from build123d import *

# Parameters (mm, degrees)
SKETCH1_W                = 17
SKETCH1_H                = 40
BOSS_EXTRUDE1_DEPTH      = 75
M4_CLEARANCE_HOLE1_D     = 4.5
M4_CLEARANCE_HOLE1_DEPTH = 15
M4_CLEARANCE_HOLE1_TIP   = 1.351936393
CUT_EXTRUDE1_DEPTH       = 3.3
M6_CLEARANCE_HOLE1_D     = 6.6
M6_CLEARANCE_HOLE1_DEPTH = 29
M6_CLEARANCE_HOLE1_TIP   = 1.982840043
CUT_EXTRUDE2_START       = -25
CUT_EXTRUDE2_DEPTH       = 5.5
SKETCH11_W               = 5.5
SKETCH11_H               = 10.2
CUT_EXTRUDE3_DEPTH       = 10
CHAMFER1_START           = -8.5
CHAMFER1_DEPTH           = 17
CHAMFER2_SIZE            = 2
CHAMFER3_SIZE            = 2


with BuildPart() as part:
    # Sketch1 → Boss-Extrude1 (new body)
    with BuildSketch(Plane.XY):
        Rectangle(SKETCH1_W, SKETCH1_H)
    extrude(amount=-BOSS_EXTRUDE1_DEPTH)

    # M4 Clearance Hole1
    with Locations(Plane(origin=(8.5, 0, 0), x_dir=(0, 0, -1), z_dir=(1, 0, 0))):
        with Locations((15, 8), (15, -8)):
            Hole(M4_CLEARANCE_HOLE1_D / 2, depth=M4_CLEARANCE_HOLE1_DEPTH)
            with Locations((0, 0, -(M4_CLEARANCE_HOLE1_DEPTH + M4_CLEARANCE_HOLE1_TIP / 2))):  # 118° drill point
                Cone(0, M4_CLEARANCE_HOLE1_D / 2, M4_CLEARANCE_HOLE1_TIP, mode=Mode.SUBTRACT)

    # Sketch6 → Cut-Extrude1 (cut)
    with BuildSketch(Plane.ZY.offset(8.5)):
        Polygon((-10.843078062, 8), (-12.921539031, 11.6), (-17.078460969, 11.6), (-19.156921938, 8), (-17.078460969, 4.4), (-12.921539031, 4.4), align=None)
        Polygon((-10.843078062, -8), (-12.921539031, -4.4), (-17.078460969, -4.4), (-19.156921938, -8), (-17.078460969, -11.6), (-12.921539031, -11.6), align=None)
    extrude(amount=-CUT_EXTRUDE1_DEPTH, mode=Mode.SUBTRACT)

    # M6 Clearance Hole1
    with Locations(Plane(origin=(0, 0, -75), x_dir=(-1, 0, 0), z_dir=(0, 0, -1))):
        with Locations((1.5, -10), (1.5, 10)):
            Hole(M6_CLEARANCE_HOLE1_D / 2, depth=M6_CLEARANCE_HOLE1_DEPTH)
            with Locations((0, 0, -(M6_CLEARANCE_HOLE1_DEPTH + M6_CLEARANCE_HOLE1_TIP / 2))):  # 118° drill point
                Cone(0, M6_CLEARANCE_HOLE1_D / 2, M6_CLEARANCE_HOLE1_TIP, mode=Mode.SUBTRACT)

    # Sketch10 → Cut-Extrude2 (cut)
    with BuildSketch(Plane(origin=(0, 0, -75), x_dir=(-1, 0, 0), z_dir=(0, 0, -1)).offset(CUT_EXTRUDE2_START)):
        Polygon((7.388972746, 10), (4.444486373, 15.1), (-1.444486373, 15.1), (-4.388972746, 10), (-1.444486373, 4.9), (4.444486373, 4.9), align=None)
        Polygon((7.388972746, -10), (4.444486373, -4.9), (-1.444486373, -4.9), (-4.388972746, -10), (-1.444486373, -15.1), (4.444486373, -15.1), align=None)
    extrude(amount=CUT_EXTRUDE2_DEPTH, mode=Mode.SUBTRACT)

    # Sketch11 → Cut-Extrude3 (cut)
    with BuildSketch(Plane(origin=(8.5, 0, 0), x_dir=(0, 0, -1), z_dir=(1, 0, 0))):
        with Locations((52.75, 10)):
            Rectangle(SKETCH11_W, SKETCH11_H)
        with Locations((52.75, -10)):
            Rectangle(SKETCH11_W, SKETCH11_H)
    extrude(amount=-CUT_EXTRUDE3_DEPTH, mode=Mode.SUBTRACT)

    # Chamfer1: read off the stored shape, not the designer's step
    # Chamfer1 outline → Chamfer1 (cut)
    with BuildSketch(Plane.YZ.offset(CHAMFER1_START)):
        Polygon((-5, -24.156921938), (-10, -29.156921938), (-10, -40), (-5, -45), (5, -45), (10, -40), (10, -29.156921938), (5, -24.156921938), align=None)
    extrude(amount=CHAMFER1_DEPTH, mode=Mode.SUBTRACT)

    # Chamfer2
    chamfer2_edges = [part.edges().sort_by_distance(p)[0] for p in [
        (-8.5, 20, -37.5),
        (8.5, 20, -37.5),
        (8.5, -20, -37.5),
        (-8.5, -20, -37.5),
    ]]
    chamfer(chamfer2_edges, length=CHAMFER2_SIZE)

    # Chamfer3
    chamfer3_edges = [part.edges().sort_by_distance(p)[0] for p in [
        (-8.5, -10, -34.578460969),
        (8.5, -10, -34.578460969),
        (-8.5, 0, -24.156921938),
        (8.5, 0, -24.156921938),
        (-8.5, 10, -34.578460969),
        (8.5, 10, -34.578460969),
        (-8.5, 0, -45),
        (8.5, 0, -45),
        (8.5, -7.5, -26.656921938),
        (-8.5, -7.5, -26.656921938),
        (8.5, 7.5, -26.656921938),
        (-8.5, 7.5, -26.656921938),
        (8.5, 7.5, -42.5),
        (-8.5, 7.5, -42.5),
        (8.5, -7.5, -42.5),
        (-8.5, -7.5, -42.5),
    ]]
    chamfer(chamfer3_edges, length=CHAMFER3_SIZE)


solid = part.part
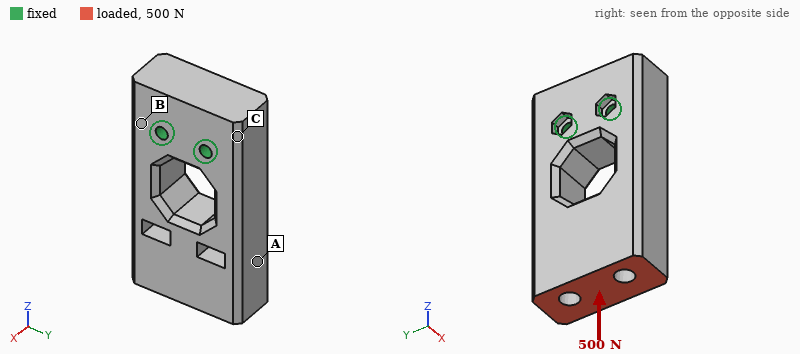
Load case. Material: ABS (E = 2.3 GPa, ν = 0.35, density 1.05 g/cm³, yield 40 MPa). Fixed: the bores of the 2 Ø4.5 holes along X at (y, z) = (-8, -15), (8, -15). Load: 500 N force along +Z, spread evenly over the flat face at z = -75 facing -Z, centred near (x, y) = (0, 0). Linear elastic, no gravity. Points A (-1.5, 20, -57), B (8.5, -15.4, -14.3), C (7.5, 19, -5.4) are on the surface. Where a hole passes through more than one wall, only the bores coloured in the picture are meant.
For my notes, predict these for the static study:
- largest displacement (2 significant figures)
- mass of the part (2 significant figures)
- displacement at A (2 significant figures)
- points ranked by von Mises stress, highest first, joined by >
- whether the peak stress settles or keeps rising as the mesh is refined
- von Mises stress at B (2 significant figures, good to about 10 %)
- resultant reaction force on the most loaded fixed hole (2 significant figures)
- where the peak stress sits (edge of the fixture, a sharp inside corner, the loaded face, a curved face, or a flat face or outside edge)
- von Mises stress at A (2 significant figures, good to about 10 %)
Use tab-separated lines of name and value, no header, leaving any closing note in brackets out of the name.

largest displacement	51 µm
mass of the part	42 g
displacement at A	31 µm
points ranked by von Mises stress, highest first, joined by >	A > B > C
whether the peak stress settles or keeps rising as the mesh is refined	keeps rising
von Mises stress at B	0.81 MPa
resultant reaction force on the most loaded fixed hole	250 N
where the peak stress sits	edge of the fixture
von Mises stress at A	1.5 MPa
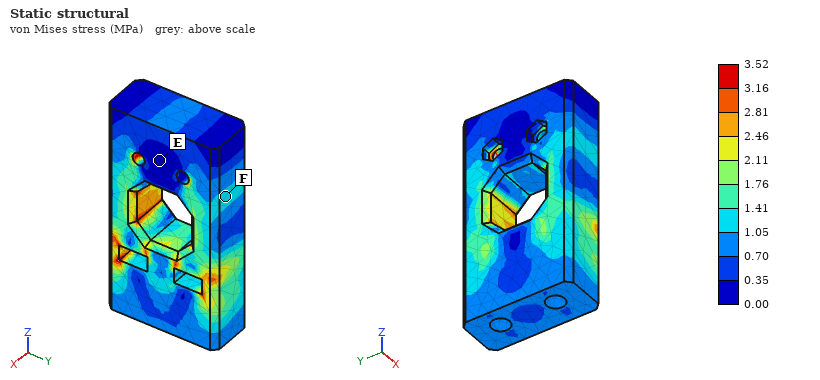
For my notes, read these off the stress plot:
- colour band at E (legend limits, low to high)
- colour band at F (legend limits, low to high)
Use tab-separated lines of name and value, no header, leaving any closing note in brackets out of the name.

colour band at E	0.00 to 0.35 MPa
colour band at F	1.05 to 1.41 MPa
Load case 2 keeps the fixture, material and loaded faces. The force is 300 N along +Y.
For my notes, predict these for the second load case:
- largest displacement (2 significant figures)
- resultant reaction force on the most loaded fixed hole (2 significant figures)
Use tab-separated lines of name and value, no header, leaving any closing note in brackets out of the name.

largest displacement	0.40 mm
resultant reaction force on the most loaded fixed hole	910 N
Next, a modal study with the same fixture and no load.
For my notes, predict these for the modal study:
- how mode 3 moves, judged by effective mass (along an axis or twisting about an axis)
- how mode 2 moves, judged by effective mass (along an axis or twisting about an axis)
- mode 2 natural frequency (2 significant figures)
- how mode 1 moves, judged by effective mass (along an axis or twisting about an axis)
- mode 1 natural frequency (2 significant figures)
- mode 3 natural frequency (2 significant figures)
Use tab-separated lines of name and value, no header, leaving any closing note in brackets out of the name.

how mode 3 moves, judged by effective mass	twisting about Z
how mode 2 moves, judged by effective mass	along Y
mode 2 natural frequency	1200 Hz
how mode 1 moves, judged by effective mass	along X
mode 1 natural frequency	770 Hz
mode 3 natural frequency	2100 Hz
